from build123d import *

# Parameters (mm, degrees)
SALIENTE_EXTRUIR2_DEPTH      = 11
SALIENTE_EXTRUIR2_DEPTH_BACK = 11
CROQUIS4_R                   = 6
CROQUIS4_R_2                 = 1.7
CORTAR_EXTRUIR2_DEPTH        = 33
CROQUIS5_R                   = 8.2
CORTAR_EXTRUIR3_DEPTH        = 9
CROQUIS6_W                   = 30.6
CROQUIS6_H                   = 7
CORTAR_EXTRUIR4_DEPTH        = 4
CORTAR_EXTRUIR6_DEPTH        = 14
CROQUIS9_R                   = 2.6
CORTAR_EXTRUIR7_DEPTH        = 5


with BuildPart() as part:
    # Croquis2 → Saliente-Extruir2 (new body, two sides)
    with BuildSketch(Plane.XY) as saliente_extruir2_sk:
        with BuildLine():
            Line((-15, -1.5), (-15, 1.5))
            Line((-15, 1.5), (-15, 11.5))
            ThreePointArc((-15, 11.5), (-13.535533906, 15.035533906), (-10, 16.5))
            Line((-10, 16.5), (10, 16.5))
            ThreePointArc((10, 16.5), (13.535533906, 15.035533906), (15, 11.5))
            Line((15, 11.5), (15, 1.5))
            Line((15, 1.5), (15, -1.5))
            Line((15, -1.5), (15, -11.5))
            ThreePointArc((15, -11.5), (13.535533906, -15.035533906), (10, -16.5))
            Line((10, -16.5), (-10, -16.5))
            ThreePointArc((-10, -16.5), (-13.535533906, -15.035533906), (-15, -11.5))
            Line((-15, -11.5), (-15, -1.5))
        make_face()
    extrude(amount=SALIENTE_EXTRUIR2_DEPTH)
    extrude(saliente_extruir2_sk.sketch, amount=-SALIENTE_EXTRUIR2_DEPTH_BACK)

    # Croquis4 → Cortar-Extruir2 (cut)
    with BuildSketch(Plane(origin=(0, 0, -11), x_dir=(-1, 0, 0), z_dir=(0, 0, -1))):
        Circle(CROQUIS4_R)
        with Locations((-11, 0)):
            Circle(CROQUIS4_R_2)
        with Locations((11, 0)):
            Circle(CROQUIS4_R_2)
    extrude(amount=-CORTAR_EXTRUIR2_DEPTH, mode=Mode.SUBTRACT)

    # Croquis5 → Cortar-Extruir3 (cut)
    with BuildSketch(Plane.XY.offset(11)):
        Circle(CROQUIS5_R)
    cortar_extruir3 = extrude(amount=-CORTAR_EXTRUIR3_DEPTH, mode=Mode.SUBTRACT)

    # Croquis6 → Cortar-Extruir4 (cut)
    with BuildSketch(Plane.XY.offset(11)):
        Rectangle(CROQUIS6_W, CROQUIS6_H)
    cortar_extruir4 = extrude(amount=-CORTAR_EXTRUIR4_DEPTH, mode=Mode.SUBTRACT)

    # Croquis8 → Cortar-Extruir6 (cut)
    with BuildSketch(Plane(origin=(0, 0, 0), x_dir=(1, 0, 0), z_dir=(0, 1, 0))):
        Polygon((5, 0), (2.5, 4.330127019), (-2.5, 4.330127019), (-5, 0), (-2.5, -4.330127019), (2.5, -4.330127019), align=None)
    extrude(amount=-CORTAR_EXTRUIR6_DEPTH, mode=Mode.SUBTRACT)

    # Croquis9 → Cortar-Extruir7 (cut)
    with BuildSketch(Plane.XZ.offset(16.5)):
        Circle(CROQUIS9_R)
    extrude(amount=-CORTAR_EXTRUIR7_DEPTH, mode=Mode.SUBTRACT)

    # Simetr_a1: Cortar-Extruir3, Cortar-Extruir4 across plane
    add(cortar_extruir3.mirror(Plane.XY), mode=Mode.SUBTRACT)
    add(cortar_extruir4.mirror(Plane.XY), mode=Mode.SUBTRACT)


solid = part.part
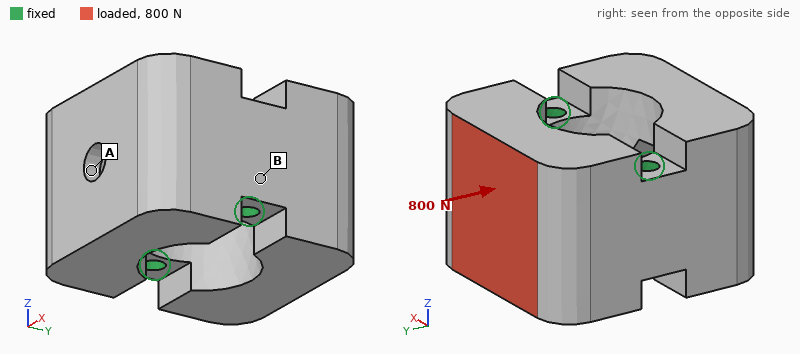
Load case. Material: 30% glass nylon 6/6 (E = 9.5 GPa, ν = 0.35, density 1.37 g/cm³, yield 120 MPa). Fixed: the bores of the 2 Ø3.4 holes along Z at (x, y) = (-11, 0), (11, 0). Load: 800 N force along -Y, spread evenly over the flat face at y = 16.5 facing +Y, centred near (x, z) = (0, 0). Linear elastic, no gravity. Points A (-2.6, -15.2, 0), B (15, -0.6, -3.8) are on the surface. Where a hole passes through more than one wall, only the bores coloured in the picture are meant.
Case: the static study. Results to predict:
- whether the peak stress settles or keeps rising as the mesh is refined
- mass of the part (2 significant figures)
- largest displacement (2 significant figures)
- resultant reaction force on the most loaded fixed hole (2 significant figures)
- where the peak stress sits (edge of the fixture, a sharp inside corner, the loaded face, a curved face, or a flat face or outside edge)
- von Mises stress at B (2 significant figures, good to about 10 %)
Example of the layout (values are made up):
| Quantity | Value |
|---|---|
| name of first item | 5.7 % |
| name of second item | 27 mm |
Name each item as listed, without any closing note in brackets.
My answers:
| Quantity | Value |
|---|---|
| whether the peak stress settles or keeps rising as the mesh is refined | keeps rising |
| mass of the part | 21 g |
| largest displacement | 8.3 µm |
| resultant reaction force on the most loaded fixed hole | 430 N |
| where the peak stress sits | edge of the fixture |
| von Mises stress at B | 1.7 MPa |
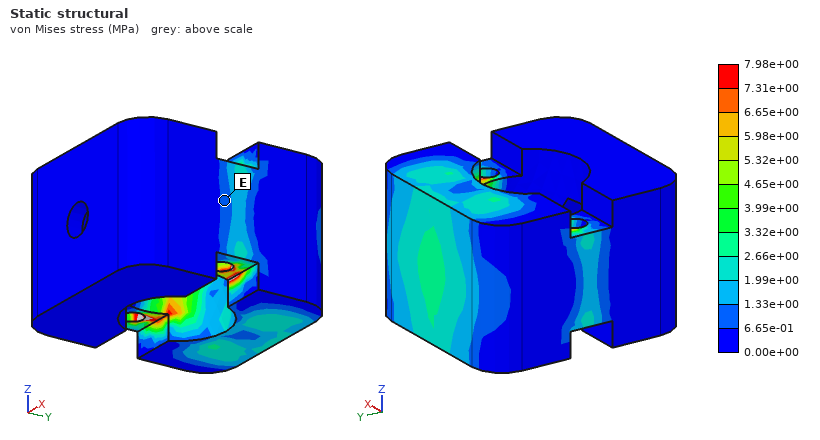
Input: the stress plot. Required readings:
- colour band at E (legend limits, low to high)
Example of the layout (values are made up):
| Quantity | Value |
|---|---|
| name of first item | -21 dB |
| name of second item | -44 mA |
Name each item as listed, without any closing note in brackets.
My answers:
| Quantity | Value |
|---|---|
| colour band at E | 6.65e-01 to 1.33e+00 MPa |
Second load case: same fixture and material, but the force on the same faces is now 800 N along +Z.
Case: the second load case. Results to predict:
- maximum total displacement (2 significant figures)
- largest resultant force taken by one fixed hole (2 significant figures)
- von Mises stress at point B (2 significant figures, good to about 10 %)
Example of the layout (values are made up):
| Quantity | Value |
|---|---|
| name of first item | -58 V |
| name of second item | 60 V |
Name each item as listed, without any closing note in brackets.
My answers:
| Quantity | Value |
|---|---|
| maximum total displacement | 55 µm |
| largest resultant force taken by one fixed hole | 400 N |
| von Mises stress at point B | 5.5 MPa |
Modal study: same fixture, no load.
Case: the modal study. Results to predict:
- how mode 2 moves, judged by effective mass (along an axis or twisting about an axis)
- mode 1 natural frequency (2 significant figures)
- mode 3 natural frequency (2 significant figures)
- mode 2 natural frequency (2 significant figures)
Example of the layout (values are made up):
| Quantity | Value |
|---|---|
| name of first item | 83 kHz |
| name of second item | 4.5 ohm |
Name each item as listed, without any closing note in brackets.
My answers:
| Quantity | Value |
|---|---|
| how mode 2 moves, judged by effective mass | along Z |
| mode 1 natural frequency | 9400 Hz |
| mode 3 natural frequency | 12 kHz |
| mode 2 natural frequency | 9900 Hz |
